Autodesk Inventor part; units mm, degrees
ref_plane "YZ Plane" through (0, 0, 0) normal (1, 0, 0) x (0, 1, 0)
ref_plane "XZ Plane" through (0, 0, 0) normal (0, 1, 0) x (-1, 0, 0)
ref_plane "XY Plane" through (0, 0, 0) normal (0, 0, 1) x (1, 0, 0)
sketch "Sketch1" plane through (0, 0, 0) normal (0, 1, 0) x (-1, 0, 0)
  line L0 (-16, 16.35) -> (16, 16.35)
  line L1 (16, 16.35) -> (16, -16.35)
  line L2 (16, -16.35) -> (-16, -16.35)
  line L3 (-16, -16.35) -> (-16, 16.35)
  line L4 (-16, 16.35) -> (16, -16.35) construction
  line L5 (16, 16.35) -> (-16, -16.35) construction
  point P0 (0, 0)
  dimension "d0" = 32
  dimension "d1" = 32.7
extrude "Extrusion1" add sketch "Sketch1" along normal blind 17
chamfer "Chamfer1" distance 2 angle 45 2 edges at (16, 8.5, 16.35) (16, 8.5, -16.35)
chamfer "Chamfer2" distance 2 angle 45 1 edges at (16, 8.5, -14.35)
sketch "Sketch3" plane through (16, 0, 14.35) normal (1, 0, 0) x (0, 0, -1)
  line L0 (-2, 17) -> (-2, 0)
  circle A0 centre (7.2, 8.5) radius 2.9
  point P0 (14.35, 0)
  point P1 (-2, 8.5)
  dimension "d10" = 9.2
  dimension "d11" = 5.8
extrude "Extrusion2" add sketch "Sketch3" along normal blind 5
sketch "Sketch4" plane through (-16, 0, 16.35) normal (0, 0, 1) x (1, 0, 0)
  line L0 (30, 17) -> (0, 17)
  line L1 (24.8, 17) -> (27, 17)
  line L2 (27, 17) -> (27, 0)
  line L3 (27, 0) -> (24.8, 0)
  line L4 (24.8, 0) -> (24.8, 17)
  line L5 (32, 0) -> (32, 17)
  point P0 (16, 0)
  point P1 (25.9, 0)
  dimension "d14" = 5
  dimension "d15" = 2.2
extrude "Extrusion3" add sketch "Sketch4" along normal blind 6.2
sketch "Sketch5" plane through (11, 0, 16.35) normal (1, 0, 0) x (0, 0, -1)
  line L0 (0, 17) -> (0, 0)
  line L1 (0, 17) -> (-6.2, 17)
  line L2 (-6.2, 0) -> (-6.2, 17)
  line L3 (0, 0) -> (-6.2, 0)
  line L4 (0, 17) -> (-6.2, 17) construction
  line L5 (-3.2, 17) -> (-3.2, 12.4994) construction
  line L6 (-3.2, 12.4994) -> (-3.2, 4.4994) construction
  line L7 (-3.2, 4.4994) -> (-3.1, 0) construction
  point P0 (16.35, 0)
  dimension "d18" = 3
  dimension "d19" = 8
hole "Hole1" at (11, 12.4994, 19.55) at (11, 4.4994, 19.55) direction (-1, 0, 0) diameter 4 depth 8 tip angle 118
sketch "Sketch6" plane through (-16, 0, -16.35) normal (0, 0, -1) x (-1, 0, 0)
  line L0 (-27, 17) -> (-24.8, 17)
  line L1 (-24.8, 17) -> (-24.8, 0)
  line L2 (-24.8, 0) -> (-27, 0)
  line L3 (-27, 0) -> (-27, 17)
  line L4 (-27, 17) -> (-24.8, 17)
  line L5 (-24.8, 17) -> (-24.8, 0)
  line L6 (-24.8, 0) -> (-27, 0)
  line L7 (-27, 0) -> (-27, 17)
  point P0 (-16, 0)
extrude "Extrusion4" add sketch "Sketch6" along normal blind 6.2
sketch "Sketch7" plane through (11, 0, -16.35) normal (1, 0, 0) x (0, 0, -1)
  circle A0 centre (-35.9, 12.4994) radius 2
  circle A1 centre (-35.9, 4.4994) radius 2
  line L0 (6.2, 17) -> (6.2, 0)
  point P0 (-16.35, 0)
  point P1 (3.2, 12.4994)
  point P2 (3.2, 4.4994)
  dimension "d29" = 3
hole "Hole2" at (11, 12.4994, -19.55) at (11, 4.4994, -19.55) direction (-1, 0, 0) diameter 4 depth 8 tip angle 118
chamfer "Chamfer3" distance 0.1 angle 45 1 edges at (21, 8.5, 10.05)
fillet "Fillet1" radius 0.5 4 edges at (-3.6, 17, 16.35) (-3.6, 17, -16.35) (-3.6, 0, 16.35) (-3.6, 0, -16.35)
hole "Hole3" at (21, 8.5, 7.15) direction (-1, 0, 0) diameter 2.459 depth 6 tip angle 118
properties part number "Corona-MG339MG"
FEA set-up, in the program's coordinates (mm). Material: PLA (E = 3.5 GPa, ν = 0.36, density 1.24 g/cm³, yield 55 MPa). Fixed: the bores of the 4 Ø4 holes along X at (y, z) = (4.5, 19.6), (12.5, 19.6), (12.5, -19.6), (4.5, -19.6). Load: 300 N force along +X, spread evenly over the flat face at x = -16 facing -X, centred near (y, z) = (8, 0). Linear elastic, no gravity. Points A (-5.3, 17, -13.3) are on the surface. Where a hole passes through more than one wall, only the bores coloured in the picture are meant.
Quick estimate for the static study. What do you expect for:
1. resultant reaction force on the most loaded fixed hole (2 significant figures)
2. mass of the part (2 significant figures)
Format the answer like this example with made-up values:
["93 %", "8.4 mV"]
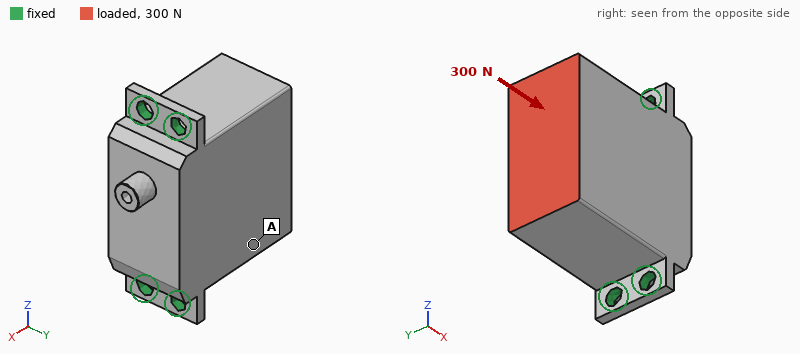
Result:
["76 N", "23 g"]
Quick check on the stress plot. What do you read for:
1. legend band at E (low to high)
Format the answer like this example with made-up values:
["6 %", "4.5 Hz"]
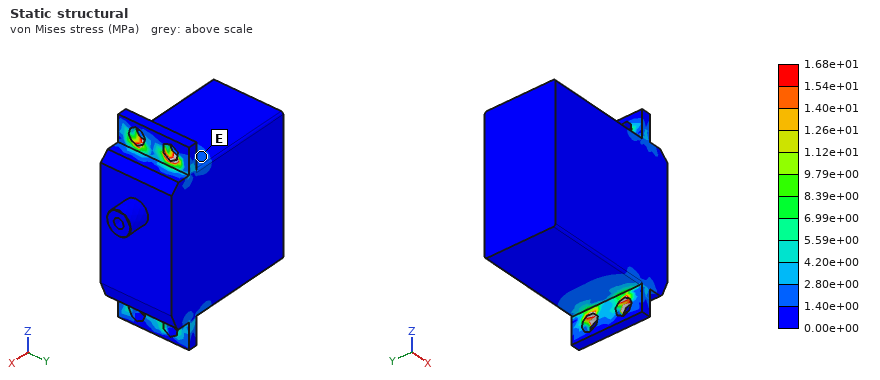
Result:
["1.40e+00 to 2.80e+00 MPa"]
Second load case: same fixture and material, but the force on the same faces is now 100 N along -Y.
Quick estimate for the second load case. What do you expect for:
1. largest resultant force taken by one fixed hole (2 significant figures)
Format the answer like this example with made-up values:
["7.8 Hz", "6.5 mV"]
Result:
["130 N"]
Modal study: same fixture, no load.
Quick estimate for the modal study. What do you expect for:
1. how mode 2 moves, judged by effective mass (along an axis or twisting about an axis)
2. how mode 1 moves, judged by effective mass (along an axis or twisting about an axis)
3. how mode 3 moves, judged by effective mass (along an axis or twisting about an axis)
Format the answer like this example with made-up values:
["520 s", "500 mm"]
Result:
["along Z", "along Y", "along X"]
